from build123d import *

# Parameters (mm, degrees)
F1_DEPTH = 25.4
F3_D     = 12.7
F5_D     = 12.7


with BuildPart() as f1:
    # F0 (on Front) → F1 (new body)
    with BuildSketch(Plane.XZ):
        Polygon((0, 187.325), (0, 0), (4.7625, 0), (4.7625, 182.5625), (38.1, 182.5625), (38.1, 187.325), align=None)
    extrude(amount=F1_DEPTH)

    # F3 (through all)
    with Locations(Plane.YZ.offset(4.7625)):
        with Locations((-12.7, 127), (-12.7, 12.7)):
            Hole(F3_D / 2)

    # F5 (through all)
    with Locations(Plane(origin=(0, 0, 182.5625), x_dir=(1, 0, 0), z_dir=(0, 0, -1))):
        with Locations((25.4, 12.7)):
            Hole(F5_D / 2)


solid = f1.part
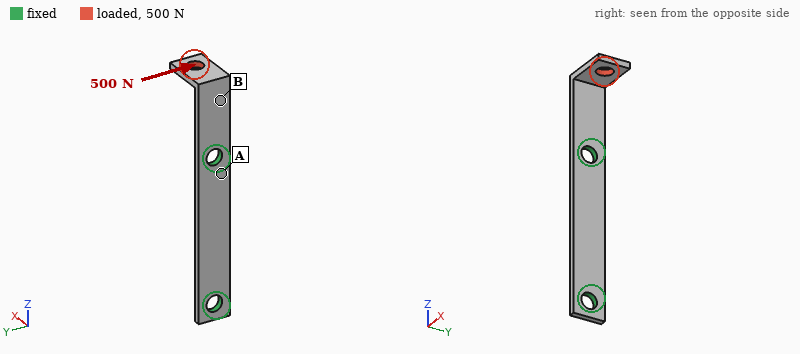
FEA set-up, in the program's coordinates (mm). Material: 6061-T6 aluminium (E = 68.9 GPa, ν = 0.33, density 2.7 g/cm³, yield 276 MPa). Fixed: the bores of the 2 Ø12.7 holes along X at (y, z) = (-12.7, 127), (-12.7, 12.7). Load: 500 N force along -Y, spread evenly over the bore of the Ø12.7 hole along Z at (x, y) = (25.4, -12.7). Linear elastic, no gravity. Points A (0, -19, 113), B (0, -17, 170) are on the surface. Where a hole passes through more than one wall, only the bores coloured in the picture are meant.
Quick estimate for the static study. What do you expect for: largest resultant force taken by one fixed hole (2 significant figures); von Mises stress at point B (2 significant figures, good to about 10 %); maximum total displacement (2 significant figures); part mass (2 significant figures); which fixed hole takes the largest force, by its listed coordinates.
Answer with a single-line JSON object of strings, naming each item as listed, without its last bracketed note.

{"largest resultant force taken by one fixed hole": "530 N", "von Mises stress at point B": "99 MPa", "maximum total displacement": "1.1 mm", "part mass": "67 g", "which fixed hole takes the largest force, by its listed coordinates": "(-12.7, 127)"}
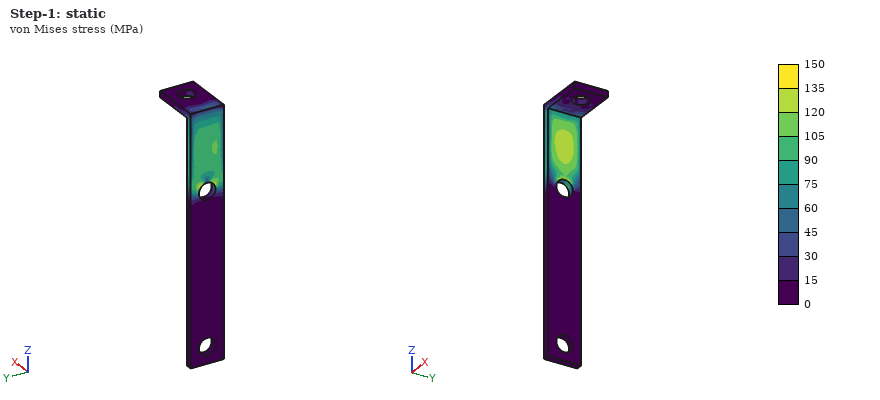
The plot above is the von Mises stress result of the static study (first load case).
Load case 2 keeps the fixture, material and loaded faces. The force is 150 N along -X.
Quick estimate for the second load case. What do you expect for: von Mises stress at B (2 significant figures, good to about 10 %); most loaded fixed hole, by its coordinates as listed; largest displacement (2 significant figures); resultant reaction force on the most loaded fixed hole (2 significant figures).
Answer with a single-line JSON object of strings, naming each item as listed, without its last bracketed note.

{"von Mises stress at B": "23 MPa", "most loaded fixed hole, by its coordinates as listed": "(-12.7, 127)", "largest displacement": "0.68 mm", "resultant reaction force on the most loaded fixed hole": "150 N"}
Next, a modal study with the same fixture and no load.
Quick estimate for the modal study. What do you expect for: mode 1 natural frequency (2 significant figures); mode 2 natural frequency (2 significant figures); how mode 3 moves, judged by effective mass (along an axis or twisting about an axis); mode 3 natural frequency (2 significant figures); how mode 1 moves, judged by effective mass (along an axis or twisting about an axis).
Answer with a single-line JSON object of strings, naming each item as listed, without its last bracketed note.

{"mode 1 natural frequency": "680 Hz", "mode 2 natural frequency": "1400 Hz", "how mode 3 moves, judged by effective mass": "along X", "mode 3 natural frequency": "2300 Hz", "how mode 1 moves, judged by effective mass": "along X"}
